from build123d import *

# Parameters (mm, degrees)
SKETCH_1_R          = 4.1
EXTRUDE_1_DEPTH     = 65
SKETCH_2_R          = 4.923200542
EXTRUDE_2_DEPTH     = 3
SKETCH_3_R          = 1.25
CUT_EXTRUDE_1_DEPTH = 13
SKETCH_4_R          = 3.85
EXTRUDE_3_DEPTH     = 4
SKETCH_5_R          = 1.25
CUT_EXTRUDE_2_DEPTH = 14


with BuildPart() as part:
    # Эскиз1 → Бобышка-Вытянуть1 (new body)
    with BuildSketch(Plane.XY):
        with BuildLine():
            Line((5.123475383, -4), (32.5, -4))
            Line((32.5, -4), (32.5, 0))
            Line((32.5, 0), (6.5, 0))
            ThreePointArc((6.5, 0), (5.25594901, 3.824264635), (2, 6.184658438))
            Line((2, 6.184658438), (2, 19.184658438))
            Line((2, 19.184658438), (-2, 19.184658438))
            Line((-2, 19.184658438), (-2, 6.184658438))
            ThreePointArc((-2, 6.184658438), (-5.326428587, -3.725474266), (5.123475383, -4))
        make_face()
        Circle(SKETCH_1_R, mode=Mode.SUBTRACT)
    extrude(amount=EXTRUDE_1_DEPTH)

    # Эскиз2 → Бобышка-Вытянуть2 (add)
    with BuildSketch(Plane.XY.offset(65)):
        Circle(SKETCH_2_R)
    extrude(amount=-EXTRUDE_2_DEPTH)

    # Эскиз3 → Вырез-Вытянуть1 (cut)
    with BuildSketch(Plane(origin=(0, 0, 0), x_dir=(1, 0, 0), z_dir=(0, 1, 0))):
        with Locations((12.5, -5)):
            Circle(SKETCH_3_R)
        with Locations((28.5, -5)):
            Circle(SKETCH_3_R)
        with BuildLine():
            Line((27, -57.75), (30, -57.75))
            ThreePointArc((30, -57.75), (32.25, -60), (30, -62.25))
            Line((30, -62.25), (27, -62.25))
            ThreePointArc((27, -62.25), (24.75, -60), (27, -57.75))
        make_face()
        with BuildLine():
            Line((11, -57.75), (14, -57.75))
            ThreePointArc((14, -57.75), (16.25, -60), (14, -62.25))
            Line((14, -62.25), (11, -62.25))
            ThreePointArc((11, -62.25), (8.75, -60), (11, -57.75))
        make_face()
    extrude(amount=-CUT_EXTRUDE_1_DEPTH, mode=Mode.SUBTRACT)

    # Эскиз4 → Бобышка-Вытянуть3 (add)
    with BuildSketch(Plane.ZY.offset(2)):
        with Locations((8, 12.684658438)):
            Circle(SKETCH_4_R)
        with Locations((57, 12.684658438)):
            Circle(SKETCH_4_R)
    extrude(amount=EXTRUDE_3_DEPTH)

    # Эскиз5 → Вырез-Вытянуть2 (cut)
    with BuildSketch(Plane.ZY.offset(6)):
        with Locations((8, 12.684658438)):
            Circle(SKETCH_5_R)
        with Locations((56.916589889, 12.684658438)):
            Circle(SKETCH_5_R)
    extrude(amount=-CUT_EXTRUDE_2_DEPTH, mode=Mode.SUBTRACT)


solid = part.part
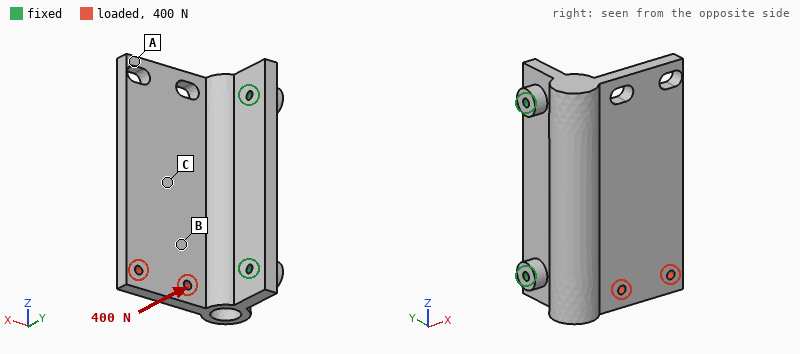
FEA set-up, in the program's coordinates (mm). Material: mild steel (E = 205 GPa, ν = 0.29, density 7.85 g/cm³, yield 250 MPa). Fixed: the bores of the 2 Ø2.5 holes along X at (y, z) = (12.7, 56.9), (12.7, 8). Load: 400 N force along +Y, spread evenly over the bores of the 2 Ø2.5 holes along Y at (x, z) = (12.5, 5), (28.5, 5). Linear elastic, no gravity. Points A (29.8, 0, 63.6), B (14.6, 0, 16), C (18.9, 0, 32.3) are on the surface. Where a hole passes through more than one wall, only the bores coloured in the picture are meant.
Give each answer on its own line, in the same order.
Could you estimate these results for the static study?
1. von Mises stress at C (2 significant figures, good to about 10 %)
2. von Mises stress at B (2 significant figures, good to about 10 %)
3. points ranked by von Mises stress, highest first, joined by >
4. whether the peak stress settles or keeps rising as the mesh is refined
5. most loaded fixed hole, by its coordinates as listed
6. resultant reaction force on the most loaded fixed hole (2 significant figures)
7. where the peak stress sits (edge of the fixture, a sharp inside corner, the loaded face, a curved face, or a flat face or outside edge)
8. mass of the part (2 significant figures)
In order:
23 MPa
36 MPa
B > C > A
keeps rising
(12.7, 8)
420 N
edge of the fixture
120 g
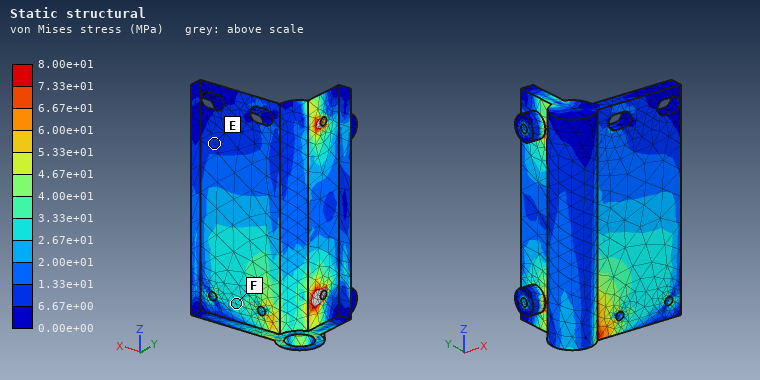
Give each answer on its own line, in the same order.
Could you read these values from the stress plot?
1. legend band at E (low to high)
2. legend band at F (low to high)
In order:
6.67e+00 to 1.33e+01 MPa
2.67e+01 to 3.33e+01 MPa
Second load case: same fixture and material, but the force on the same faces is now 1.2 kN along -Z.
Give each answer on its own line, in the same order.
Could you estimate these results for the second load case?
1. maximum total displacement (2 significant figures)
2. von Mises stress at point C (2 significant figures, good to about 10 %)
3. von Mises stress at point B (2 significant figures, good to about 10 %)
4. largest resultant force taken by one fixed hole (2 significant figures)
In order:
17 µm
12 MPa
13 MPa
850 N
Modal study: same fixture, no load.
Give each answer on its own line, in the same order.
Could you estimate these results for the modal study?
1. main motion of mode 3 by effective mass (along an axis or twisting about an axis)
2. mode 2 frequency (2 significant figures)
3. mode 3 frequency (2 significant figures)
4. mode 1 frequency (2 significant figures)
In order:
along X
4800 Hz
6300 Hz
1800 Hz
